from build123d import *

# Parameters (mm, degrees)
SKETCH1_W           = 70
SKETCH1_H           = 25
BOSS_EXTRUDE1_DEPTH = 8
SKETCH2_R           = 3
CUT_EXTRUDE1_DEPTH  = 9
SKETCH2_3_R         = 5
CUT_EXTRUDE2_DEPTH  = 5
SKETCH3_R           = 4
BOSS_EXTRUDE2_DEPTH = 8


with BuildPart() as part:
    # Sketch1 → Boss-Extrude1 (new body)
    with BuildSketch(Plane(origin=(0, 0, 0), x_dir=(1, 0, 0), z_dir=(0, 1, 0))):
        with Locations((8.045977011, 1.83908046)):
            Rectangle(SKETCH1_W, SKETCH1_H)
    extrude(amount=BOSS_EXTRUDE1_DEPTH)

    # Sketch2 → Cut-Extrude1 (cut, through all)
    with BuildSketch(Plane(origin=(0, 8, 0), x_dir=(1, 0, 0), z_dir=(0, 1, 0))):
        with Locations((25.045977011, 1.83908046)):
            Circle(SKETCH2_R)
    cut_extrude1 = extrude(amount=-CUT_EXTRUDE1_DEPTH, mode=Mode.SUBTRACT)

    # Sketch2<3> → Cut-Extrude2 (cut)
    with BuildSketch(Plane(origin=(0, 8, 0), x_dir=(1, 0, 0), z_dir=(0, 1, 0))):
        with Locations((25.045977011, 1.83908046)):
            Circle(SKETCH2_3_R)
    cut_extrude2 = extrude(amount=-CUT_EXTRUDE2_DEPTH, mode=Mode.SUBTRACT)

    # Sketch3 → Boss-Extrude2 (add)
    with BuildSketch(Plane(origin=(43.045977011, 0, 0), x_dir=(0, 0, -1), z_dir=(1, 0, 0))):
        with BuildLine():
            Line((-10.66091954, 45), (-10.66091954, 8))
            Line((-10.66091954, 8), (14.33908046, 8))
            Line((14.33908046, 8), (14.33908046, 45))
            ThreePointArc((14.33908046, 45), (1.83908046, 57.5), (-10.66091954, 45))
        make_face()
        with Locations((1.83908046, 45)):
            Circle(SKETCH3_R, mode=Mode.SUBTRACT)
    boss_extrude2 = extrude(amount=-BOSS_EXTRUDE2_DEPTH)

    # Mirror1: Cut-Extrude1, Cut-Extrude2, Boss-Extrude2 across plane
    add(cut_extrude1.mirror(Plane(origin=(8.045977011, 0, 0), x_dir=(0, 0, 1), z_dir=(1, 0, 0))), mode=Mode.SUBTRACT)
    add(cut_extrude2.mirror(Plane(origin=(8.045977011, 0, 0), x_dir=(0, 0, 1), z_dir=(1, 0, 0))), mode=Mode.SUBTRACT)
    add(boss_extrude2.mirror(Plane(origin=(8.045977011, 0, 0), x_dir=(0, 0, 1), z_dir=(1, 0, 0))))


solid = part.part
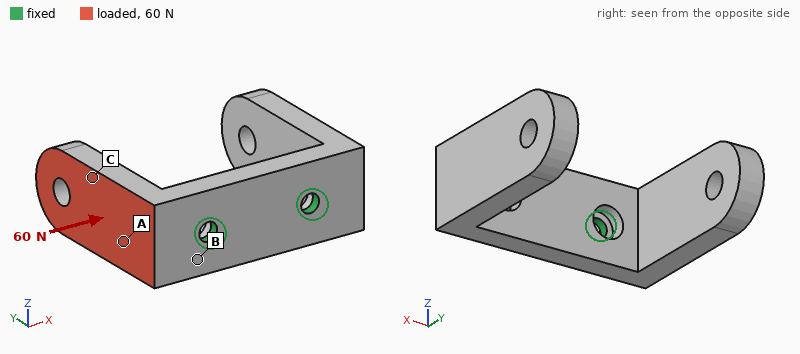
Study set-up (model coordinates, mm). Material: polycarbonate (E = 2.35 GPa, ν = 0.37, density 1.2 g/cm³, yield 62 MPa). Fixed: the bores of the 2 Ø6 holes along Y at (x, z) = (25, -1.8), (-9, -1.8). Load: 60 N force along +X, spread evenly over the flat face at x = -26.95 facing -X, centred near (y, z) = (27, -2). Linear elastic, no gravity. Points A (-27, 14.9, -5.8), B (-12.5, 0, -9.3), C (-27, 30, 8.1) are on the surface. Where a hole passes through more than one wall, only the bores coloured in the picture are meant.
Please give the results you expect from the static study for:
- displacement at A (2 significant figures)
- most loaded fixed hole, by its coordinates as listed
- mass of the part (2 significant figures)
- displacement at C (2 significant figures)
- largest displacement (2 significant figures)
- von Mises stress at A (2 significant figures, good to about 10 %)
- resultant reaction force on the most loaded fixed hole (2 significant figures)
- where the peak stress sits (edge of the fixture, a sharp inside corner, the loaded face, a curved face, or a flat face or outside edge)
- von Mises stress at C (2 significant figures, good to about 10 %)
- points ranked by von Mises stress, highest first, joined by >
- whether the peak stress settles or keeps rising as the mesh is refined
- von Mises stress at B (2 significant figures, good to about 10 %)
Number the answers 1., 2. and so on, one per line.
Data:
1. 0.23 mm
2. (25, -1.8)
3. 37 g
4. 0.45 mm
5. 0.97 mm
6. 3.0 MPa
7. 100 N
8. edge of the fixture
9. 1.3 MPa
10. B > A > C
11. keeps rising
12. 5.0 MPa
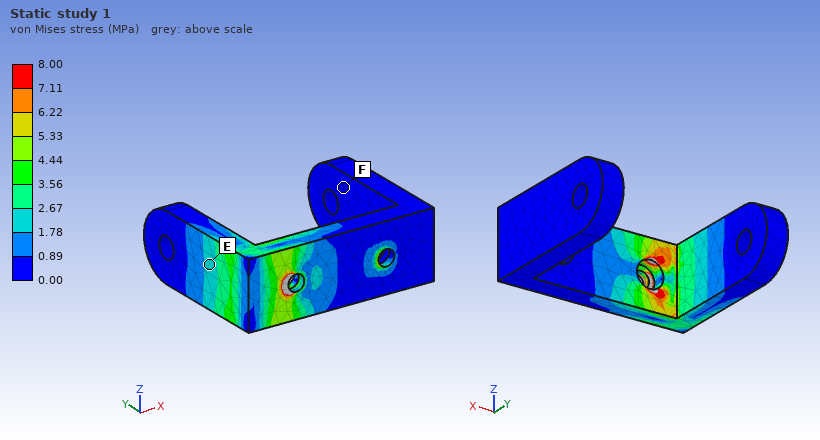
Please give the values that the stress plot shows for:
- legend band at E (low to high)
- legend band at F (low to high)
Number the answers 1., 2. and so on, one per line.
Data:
1. 1.78 to 2.67 MPa
2. 0.00 to 0.89 MPa
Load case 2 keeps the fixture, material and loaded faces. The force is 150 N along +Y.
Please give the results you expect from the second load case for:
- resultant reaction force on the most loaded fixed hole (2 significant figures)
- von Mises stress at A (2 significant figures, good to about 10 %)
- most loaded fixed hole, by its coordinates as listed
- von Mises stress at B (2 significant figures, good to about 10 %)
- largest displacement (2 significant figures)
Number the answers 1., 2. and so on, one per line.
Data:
1. 250 N
2. 2.2 MPa
3. (-9, -1.8)
4. 7.2 MPa
5. 1.1 mm
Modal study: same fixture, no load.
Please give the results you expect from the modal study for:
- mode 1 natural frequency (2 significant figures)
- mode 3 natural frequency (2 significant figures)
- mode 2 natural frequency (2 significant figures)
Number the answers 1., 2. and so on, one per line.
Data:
1. 440 Hz
2. 460 Hz
3. 440 Hz
